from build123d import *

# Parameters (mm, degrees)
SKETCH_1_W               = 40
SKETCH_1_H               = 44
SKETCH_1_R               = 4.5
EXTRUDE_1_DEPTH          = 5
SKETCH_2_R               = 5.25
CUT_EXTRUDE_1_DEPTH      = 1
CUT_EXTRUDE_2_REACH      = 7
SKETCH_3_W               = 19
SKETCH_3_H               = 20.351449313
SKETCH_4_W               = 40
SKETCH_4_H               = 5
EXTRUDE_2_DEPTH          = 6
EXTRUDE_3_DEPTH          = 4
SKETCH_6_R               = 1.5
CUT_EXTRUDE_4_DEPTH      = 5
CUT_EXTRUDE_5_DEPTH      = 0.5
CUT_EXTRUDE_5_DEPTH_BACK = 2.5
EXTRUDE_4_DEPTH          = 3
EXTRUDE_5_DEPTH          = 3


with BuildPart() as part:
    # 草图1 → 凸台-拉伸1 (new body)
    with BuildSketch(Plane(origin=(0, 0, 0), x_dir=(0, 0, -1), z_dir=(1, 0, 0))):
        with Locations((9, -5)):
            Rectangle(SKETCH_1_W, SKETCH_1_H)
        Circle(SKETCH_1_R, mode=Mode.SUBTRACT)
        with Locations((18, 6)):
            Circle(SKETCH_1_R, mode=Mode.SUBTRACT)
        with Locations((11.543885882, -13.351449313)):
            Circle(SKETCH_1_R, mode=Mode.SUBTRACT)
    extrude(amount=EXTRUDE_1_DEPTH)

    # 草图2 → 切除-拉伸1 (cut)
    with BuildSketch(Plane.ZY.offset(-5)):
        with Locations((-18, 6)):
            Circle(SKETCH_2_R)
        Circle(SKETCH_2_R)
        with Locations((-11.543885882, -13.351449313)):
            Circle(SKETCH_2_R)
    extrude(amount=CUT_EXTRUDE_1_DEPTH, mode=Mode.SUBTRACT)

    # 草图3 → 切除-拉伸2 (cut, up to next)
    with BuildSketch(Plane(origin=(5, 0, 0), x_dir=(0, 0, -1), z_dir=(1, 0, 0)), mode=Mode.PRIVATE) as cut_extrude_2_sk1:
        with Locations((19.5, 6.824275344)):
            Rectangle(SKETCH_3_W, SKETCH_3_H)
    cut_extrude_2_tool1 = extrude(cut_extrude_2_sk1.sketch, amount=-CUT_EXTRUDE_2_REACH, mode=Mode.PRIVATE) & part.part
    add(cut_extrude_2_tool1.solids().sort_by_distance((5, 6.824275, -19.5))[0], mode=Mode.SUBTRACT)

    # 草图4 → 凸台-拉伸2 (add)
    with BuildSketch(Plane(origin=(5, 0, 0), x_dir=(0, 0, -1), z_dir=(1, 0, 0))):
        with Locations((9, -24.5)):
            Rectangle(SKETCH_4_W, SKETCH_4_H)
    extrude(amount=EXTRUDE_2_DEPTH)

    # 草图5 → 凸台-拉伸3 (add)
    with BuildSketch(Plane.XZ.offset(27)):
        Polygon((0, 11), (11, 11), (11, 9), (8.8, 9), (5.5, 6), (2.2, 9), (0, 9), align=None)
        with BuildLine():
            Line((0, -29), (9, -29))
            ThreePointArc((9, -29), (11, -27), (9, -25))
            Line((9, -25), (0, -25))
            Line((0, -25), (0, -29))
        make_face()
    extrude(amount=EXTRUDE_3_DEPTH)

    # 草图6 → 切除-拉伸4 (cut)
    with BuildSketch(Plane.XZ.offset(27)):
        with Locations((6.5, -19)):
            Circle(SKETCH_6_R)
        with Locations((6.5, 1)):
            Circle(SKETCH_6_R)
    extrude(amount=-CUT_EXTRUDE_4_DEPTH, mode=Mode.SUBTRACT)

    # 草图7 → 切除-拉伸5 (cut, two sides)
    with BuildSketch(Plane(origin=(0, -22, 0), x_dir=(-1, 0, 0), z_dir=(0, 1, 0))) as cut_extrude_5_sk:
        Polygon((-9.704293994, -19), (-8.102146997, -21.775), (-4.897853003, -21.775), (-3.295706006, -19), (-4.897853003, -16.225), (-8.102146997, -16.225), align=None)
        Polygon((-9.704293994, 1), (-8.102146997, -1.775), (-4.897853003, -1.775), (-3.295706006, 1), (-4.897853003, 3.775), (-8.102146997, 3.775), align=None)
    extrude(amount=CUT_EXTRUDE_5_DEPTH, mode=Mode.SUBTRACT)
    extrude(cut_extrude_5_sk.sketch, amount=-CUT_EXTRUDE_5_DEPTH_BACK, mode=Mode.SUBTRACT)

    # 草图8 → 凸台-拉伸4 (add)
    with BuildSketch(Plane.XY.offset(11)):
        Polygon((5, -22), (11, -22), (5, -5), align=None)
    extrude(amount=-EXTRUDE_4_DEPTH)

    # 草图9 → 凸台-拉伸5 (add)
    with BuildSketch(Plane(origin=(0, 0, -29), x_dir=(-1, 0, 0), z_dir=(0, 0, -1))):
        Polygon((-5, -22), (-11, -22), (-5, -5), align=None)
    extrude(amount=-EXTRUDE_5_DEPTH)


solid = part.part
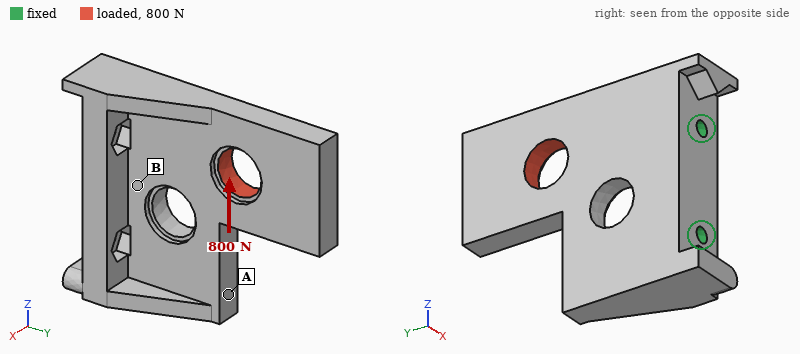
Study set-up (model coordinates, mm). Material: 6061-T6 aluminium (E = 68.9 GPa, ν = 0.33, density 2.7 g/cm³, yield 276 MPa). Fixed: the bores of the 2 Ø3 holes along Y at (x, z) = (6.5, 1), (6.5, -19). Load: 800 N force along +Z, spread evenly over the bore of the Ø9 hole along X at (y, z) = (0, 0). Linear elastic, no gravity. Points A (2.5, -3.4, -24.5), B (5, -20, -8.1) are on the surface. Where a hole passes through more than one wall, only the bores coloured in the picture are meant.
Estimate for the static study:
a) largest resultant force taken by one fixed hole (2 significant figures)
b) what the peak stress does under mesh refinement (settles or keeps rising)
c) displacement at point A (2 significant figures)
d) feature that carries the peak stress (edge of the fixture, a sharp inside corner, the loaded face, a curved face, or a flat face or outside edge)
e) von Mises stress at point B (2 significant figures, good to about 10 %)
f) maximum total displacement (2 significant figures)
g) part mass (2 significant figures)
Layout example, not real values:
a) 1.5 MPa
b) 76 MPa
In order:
a) 1.1 kN
b) keeps rising
c) 33 µm
d) edge of the fixture
e) 40 MPa
f) 72 µm
g) 21 g
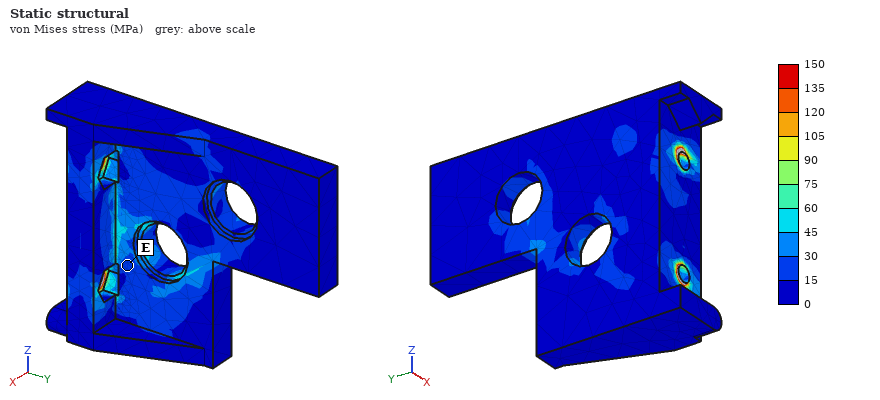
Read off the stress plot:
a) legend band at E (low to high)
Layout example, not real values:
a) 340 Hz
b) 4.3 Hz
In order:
a) 15 to 30 MPa
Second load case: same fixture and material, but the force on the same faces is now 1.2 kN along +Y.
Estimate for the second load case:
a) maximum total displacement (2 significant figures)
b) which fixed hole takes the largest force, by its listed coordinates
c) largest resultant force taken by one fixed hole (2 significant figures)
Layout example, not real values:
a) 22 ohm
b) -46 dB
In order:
a) 0.14 mm
b) (6.5, 1)
c) 1.1 kN
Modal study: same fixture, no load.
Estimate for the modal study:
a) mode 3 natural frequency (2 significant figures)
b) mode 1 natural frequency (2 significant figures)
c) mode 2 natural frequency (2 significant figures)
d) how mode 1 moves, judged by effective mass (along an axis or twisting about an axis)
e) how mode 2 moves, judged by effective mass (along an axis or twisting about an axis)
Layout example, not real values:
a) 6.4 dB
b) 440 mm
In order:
a) 7600 Hz
b) 2000 Hz
c) 5800 Hz
d) along X
e) along Z
